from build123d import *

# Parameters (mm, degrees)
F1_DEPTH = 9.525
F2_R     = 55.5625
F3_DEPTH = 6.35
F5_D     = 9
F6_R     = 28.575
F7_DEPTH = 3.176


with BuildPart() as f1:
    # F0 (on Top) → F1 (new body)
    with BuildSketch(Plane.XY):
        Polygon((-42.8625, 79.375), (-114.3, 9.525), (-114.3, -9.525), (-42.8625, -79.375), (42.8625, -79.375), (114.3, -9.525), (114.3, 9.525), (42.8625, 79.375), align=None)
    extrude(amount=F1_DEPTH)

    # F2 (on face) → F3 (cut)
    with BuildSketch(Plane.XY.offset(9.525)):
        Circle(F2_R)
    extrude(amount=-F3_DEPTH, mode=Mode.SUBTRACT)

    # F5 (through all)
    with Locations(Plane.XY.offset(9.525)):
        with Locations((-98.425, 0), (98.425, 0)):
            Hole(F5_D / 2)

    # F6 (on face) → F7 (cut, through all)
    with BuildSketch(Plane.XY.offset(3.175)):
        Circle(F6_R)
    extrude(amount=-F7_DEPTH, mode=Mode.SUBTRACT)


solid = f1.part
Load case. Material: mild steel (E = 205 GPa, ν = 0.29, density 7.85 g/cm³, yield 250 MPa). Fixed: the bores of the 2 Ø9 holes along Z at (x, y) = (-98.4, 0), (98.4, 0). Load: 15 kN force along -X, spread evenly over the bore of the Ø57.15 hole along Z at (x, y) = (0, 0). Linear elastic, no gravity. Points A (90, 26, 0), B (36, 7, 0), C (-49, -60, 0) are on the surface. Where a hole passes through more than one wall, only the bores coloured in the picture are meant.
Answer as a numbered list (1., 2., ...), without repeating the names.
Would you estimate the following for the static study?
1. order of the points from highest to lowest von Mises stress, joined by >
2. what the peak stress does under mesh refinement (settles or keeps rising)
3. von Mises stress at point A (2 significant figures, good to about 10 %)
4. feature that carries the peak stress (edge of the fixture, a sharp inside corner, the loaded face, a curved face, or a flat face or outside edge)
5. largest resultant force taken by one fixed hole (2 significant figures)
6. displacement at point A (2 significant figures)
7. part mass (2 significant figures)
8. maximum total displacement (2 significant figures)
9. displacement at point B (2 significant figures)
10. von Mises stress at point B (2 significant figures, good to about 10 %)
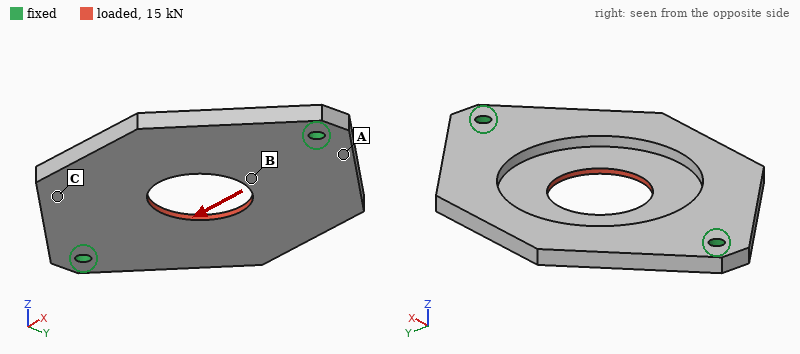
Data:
1. B > A > C
2. keeps rising
3. 12 MPa
4. edge of the fixture
5. 7.5 kN
6. 3.8 µm
7. 1.4 kg
8. 17 µm
9. 15 µm
10. 32 MPa
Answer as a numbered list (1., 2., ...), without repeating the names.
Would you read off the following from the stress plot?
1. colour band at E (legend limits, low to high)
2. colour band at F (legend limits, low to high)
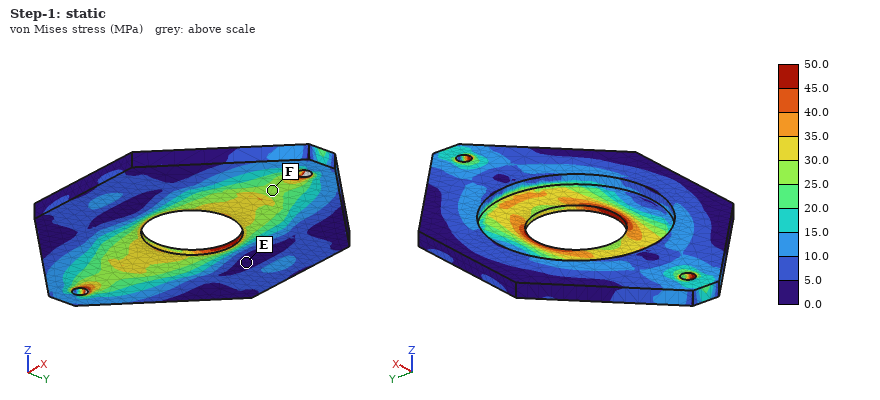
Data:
1. 0.0 to 5.0 MPa
2. 25.0 to 30.0 MPa
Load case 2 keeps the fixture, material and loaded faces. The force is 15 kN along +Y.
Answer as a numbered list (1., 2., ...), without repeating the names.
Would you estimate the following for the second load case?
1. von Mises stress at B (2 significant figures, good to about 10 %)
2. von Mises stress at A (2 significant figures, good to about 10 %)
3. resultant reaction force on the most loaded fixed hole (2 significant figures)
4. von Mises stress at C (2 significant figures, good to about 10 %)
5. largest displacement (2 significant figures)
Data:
1. 27 MPa
2. 33 MPa
3. 7.5 kN
4. 17 MPa
5. 81 µm
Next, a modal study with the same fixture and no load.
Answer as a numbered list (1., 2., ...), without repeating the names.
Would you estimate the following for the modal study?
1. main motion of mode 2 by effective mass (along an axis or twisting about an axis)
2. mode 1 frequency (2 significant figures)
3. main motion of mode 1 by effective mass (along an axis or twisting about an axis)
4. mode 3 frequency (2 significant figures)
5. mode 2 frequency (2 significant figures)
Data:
1. along Z
2. 700 Hz
3. twisting about X
4. 1900 Hz
5. 840 Hz
